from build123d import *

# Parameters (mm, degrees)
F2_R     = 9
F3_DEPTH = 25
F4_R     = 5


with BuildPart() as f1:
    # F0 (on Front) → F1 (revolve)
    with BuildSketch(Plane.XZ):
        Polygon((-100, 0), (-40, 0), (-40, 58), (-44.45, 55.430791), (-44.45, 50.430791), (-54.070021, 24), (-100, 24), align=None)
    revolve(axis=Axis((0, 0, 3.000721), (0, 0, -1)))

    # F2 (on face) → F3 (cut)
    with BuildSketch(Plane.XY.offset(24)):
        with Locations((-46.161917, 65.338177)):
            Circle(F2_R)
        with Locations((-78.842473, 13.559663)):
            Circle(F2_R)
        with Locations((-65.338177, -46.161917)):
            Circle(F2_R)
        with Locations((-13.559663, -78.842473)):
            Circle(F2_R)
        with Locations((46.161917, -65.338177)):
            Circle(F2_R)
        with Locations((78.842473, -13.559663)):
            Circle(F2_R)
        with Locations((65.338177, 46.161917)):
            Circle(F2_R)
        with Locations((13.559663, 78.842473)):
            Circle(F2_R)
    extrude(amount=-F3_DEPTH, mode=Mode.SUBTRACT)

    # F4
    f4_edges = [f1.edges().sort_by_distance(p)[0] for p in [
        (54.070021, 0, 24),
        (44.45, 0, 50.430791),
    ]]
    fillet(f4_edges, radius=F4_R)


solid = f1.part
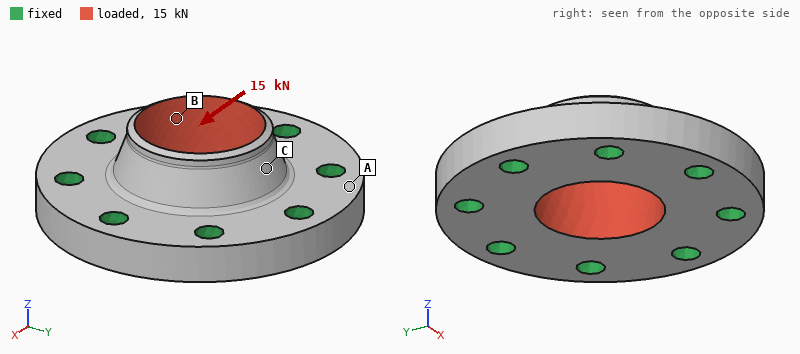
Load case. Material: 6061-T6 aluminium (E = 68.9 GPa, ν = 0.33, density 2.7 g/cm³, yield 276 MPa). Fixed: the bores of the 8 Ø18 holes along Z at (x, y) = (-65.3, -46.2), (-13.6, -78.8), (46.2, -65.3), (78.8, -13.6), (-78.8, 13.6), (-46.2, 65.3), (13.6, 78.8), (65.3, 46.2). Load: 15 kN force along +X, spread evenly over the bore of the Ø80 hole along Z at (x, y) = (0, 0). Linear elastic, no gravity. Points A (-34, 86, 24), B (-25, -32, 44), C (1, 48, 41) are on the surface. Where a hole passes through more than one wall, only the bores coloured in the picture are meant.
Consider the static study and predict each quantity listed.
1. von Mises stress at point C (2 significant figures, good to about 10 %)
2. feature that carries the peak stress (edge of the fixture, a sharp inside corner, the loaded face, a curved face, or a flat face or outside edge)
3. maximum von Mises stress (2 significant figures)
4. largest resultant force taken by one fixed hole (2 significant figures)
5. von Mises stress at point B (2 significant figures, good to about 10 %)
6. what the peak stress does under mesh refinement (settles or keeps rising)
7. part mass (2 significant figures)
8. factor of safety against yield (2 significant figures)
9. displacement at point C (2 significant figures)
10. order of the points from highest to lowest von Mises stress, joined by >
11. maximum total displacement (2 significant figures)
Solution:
4.1 MPa
the loaded face
13 MPa
2.8 kN
7.1 MPa
settles
1.8 kg
21
3.5 µm
B > C > A
13 µm
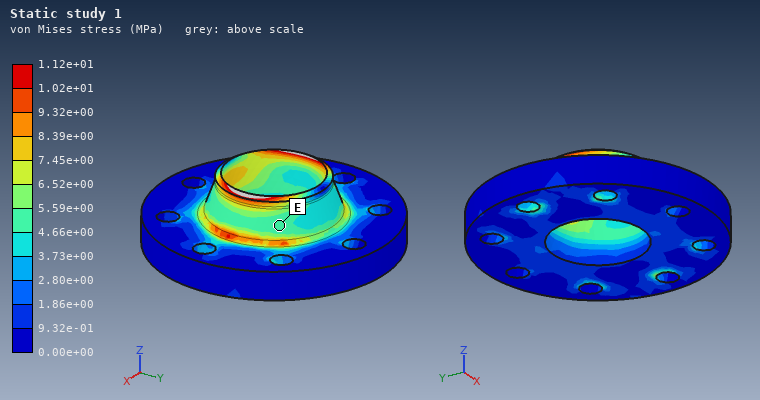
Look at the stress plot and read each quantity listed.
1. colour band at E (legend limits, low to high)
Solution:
4.66e+00 to 5.59e+00 MPa
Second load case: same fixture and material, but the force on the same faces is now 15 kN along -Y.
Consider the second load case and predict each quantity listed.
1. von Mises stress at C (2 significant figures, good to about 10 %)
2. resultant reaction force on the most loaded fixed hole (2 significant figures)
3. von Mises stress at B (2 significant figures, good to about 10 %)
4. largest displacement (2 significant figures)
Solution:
5.4 MPa
2.8 kN
6.3 MPa
13 µm
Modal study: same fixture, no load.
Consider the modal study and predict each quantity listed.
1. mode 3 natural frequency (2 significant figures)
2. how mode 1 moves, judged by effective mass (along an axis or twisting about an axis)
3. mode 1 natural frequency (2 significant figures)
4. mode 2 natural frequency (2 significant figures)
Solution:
14 kHz
along Z
11 kHz
14 kHz
